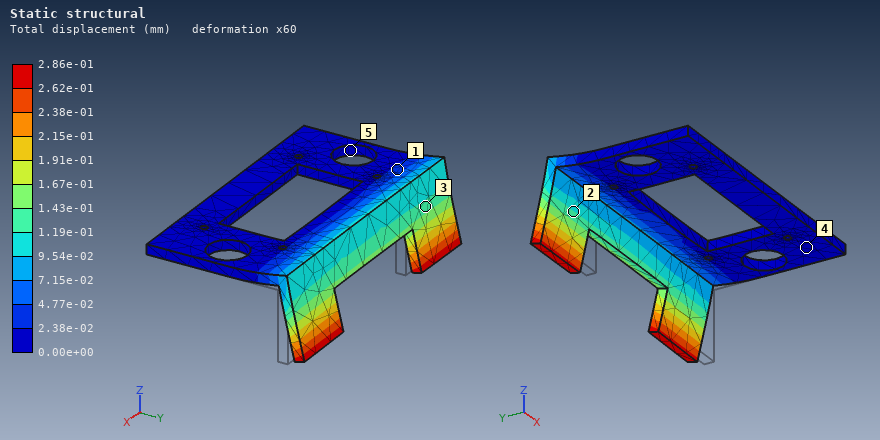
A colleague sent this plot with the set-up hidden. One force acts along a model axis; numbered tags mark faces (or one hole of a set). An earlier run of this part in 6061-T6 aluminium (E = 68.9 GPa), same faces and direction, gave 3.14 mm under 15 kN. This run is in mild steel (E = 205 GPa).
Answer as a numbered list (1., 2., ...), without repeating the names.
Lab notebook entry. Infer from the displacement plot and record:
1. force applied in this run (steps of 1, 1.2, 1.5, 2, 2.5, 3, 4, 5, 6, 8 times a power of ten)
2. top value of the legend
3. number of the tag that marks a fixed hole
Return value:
1. 4 kN
2. 2.86e-01 mm
3. 5
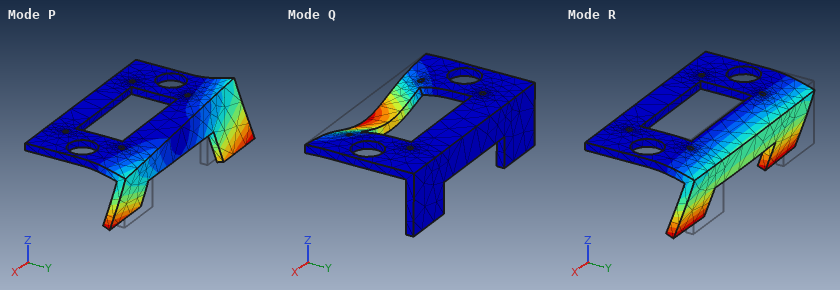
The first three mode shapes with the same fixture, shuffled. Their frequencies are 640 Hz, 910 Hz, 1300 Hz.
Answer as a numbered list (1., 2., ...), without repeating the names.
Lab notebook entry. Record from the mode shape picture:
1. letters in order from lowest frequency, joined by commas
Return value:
1. R, P, Q
